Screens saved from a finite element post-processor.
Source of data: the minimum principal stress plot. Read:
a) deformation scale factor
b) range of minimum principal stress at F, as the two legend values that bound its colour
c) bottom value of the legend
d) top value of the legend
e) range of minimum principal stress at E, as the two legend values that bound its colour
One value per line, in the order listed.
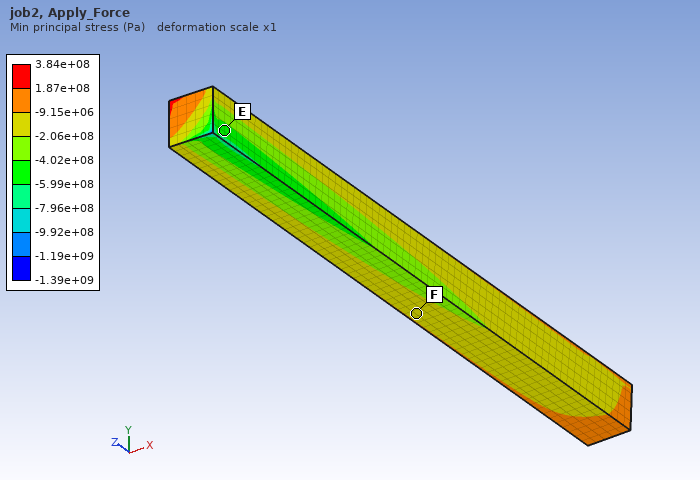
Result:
1
-2.06e+08 to -9.15e+06 Pa
-1.39e+09 Pa
3.84e+08 Pa
-5.99e+08 to -4.02e+08 Pa
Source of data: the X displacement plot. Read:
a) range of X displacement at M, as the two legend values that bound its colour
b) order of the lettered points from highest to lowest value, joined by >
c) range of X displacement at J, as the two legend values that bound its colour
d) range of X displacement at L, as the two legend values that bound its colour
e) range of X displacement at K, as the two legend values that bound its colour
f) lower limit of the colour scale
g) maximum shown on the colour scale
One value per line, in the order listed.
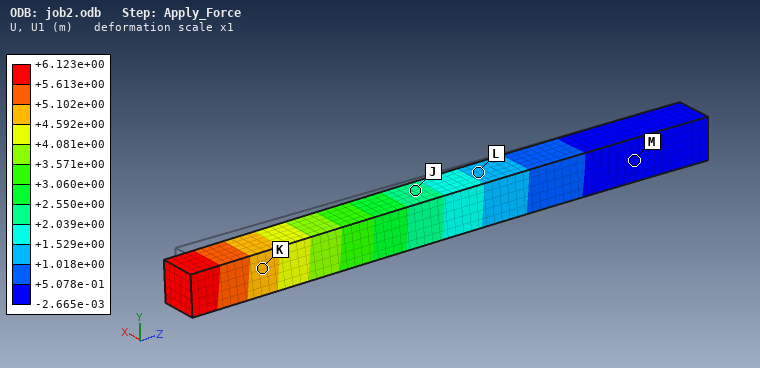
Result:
-2.665e-03 to +5.078e-01 m
K > J > L > M
+2.039e+00 to +2.550e+00 m
+1.018e+00 to +1.529e+00 m
+4.592e+00 to +5.102e+00 m
-2.665e-03 m
+6.123e+00 m
